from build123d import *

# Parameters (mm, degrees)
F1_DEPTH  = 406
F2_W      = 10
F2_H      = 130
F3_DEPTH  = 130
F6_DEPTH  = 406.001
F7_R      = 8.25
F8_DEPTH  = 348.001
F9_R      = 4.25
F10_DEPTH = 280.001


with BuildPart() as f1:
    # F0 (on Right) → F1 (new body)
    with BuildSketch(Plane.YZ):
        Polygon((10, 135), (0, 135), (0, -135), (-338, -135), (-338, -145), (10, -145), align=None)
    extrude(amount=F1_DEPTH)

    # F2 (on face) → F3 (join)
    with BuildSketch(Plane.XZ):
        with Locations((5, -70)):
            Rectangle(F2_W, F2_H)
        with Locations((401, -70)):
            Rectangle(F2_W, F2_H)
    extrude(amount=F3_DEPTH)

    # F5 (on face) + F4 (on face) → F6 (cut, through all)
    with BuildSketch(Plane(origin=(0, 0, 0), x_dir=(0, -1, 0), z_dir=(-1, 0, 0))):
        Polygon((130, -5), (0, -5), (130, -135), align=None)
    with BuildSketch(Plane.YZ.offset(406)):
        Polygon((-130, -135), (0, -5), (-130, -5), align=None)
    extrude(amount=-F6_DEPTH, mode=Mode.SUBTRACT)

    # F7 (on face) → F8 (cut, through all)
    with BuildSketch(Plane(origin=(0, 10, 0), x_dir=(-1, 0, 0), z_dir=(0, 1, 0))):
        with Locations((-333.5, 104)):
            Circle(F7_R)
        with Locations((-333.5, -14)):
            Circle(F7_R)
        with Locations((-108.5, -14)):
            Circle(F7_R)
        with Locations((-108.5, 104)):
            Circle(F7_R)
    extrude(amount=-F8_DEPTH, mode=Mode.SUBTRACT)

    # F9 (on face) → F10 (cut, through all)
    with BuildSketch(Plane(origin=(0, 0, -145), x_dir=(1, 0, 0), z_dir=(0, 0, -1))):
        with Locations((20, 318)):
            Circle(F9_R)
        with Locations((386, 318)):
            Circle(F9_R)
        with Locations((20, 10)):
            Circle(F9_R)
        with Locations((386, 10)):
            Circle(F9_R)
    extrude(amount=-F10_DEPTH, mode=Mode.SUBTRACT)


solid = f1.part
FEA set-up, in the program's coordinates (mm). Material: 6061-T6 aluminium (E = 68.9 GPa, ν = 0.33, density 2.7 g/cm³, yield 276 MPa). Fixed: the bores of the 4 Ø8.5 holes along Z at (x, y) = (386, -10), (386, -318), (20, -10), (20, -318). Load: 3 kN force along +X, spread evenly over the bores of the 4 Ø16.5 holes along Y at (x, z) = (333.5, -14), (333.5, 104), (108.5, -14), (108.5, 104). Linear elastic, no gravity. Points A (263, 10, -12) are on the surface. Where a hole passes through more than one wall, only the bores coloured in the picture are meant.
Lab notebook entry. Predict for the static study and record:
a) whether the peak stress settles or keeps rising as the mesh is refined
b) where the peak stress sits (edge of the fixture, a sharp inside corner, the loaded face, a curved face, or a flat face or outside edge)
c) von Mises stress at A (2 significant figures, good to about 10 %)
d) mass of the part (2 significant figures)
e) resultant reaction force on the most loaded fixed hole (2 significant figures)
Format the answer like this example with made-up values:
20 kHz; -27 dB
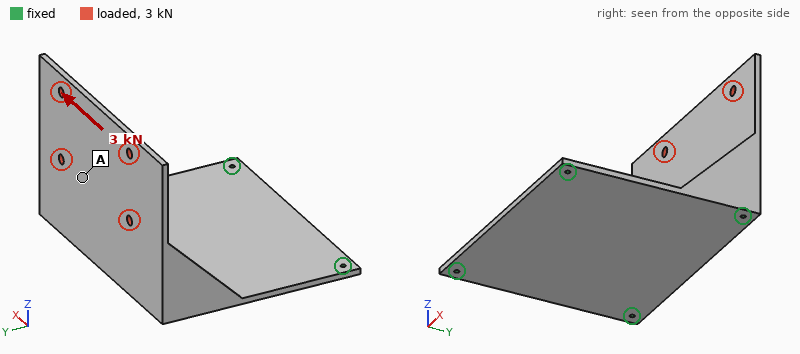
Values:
keeps rising; edge of the fixture; 0.81 MPa; 7.2 kg; 2.0 kN
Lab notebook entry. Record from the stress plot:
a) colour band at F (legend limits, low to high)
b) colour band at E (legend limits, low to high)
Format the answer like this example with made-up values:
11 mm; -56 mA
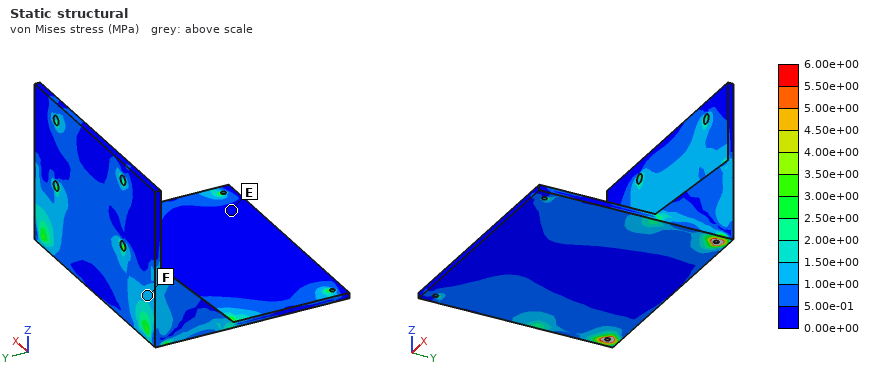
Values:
1.00e+00 to 1.50e+00 MPa; 0.00e+00 to 5.00e-01 MPa
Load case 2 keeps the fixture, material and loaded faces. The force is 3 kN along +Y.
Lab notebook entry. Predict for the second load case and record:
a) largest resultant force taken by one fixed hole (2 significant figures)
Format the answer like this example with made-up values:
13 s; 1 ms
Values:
1.4 kN
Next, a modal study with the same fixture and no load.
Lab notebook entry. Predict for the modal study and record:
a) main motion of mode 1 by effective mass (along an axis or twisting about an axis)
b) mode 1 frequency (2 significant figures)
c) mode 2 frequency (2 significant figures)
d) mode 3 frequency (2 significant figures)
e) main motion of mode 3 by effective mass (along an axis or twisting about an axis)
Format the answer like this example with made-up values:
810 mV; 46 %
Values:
along Y; 130 Hz; 280 Hz; 320 Hz; along Z
